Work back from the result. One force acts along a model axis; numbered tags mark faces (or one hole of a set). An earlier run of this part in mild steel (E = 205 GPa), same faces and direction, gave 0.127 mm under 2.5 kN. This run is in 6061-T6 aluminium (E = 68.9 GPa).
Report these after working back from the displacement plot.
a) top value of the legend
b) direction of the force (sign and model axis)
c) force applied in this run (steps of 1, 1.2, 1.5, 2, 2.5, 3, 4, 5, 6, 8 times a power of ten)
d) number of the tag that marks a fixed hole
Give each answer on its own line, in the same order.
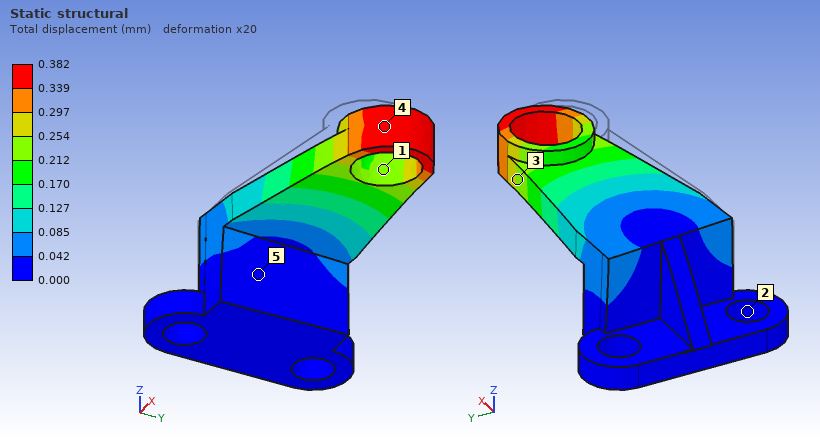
0.382 mm
+Y
2.5 kN
2
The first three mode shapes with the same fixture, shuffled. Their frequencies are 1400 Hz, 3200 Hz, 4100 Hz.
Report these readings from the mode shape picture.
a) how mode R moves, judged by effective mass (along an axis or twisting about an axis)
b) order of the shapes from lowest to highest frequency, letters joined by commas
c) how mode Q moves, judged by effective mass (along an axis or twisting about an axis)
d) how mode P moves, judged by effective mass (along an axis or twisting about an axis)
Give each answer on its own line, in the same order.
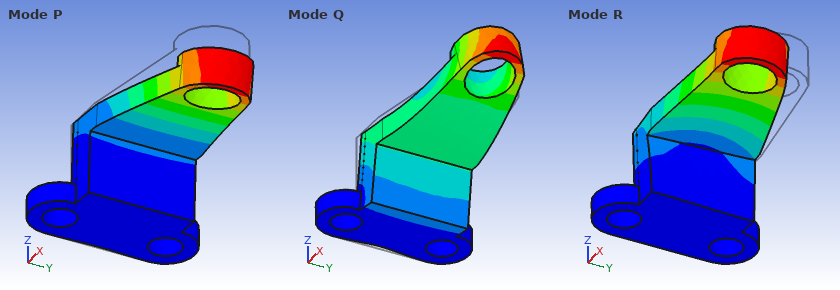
along Y
P, R, Q
along X
along Z
